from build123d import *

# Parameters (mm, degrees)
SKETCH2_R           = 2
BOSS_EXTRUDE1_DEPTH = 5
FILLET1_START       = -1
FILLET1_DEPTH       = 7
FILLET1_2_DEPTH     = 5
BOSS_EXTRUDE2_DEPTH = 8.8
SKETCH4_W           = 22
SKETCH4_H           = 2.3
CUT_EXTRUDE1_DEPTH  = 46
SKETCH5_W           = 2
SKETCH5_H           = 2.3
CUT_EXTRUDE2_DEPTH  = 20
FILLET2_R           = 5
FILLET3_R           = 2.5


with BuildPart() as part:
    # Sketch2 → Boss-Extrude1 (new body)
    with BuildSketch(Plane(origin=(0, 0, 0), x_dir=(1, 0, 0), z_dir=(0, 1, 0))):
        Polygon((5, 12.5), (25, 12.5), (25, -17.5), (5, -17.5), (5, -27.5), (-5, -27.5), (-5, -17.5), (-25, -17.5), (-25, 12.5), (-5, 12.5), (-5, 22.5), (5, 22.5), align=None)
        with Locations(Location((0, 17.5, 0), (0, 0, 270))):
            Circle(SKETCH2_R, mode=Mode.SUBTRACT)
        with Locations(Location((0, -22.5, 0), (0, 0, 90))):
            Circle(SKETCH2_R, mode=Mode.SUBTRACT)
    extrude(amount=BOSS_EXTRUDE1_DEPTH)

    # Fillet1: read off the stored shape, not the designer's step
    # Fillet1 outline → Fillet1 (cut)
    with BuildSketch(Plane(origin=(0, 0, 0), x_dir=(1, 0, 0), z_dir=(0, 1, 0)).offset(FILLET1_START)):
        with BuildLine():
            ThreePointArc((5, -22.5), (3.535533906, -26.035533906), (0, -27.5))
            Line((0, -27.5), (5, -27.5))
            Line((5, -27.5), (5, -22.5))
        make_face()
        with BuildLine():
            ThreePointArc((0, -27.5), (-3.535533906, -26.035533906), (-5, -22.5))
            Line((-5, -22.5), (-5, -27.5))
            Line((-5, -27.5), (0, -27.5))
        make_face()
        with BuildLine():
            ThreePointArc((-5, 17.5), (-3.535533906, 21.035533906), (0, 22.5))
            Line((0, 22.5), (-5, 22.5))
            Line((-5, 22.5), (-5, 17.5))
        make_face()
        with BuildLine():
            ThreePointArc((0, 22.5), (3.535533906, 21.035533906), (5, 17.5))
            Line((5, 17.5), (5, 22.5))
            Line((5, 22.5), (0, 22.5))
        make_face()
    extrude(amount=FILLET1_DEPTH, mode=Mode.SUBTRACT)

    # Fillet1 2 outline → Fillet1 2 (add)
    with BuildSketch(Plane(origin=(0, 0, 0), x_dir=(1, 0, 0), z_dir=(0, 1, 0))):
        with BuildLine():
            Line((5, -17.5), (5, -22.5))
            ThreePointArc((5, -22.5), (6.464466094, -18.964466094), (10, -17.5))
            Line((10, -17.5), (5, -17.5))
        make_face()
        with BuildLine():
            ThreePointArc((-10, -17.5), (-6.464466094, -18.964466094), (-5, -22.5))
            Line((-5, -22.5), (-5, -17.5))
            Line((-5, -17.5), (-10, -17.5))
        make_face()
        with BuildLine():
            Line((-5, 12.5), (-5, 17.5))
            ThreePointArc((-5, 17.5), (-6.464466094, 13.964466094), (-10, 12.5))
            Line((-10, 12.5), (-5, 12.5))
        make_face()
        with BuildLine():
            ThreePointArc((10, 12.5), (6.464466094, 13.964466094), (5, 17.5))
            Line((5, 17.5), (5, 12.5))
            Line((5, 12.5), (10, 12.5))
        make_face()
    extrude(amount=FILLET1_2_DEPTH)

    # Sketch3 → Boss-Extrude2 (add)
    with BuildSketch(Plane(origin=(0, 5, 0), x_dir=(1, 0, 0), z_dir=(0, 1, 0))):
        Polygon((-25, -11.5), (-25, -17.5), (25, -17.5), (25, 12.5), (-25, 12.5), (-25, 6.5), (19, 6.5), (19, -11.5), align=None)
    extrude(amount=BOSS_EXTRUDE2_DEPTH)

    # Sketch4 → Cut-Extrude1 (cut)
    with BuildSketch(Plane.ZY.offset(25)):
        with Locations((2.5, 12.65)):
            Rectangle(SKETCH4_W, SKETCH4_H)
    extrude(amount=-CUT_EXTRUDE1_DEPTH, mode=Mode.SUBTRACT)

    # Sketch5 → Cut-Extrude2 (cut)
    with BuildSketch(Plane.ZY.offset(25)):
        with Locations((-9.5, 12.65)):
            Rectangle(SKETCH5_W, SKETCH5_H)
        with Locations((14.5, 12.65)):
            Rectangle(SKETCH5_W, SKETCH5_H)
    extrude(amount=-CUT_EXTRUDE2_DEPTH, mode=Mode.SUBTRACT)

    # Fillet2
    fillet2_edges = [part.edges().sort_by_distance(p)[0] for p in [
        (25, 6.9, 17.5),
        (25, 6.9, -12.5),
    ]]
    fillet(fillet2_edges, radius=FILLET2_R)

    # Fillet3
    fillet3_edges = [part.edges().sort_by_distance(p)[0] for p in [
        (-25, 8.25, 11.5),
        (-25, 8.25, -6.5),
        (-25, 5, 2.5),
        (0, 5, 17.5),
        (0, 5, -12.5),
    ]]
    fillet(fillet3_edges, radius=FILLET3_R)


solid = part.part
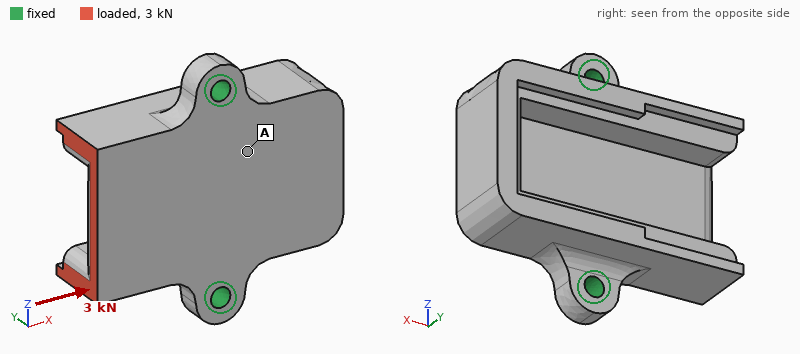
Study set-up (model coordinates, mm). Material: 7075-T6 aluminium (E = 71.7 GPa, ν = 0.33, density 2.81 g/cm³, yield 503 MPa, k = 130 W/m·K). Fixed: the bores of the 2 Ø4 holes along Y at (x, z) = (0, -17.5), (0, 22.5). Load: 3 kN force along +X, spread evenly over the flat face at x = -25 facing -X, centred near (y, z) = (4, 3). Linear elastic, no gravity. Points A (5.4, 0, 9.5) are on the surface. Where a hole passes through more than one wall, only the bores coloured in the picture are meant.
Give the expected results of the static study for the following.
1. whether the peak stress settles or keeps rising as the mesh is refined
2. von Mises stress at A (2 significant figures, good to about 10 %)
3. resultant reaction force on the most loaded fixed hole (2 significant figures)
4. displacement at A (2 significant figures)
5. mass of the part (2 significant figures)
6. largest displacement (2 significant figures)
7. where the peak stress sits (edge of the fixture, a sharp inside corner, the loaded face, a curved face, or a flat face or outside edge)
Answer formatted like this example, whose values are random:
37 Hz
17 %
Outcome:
keeps rising
12 MPa
1.5 kN
7.8 µm
39 g
38 µm
edge of the fixture
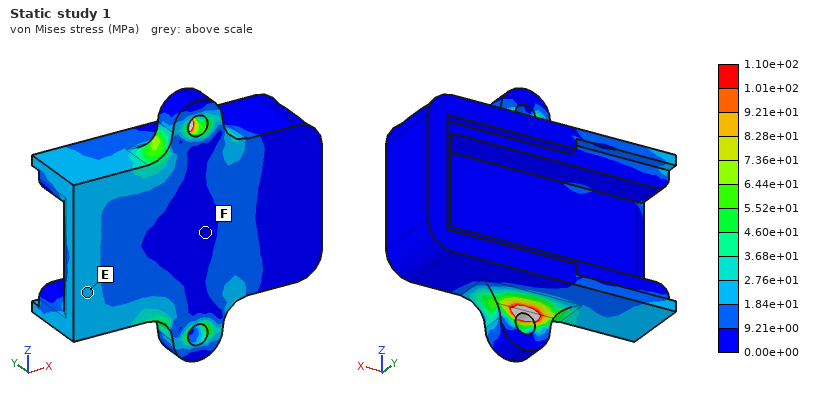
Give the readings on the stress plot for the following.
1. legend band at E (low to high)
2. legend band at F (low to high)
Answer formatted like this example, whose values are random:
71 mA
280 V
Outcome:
1.84e+01 to 2.76e+01 MPa
0.00e+00 to 9.21e+00 MPa
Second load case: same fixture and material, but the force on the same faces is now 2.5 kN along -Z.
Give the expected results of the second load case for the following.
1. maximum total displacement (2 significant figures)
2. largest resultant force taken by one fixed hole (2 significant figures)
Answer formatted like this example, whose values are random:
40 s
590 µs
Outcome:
59 µm
2.1 kN
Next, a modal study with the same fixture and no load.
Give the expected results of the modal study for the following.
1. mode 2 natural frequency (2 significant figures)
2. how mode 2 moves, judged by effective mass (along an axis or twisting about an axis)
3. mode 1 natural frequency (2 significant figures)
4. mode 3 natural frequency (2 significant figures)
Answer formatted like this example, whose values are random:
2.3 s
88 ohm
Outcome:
8300 Hz
along Y
3600 Hz
11 kHz
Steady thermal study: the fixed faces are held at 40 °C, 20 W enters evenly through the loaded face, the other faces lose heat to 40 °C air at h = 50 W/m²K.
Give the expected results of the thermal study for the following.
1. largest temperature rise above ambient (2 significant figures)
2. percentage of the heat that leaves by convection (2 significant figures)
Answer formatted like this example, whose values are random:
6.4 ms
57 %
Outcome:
22 K
14 %
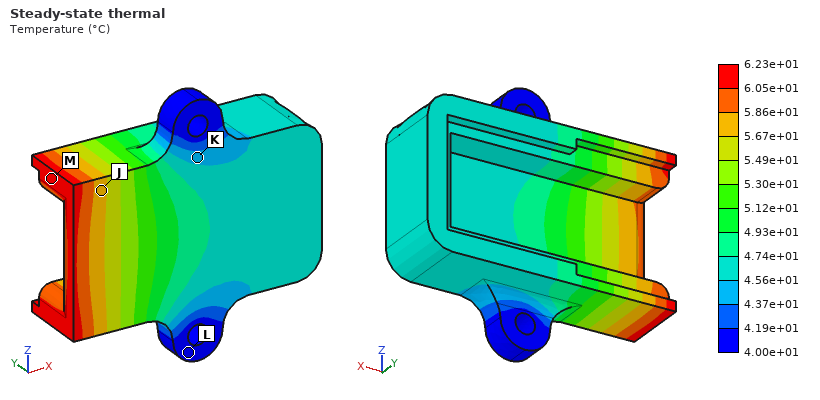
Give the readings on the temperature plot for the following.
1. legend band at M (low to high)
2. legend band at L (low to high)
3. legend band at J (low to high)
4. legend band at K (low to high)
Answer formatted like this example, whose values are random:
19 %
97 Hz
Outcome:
6.05e+01 to 6.23e+01 °C
4.00e+01 to 4.19e+01 °C
5.67e+01 to 5.86e+01 °C
4.37e+01 to 4.56e+01 °C
